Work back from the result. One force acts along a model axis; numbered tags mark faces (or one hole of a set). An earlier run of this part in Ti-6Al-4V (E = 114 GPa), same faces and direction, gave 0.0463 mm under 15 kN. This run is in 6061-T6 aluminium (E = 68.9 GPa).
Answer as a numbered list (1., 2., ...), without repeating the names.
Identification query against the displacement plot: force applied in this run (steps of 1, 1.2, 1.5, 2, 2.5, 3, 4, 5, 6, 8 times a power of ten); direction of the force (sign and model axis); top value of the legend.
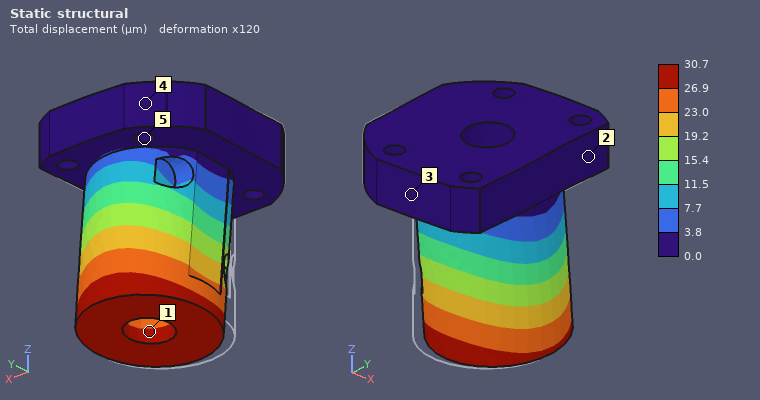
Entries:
1. 6 kN
2. +Y
3. 30.7 µm
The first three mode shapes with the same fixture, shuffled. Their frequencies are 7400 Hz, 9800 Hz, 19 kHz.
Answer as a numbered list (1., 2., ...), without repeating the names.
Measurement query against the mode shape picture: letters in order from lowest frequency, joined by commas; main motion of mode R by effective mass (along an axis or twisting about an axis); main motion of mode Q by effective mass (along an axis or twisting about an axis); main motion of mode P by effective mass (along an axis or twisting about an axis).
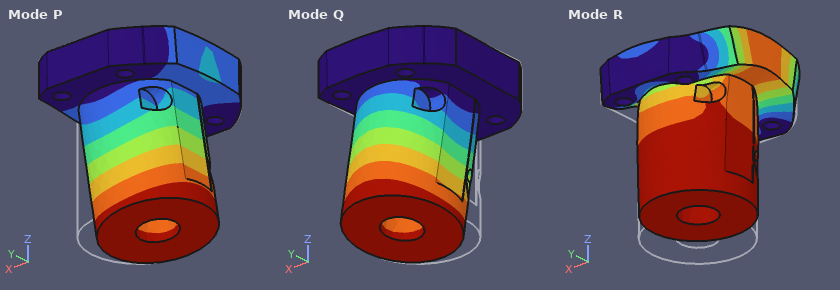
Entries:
1. P, Q, R
2. along Z
3. along Y
4. along X
